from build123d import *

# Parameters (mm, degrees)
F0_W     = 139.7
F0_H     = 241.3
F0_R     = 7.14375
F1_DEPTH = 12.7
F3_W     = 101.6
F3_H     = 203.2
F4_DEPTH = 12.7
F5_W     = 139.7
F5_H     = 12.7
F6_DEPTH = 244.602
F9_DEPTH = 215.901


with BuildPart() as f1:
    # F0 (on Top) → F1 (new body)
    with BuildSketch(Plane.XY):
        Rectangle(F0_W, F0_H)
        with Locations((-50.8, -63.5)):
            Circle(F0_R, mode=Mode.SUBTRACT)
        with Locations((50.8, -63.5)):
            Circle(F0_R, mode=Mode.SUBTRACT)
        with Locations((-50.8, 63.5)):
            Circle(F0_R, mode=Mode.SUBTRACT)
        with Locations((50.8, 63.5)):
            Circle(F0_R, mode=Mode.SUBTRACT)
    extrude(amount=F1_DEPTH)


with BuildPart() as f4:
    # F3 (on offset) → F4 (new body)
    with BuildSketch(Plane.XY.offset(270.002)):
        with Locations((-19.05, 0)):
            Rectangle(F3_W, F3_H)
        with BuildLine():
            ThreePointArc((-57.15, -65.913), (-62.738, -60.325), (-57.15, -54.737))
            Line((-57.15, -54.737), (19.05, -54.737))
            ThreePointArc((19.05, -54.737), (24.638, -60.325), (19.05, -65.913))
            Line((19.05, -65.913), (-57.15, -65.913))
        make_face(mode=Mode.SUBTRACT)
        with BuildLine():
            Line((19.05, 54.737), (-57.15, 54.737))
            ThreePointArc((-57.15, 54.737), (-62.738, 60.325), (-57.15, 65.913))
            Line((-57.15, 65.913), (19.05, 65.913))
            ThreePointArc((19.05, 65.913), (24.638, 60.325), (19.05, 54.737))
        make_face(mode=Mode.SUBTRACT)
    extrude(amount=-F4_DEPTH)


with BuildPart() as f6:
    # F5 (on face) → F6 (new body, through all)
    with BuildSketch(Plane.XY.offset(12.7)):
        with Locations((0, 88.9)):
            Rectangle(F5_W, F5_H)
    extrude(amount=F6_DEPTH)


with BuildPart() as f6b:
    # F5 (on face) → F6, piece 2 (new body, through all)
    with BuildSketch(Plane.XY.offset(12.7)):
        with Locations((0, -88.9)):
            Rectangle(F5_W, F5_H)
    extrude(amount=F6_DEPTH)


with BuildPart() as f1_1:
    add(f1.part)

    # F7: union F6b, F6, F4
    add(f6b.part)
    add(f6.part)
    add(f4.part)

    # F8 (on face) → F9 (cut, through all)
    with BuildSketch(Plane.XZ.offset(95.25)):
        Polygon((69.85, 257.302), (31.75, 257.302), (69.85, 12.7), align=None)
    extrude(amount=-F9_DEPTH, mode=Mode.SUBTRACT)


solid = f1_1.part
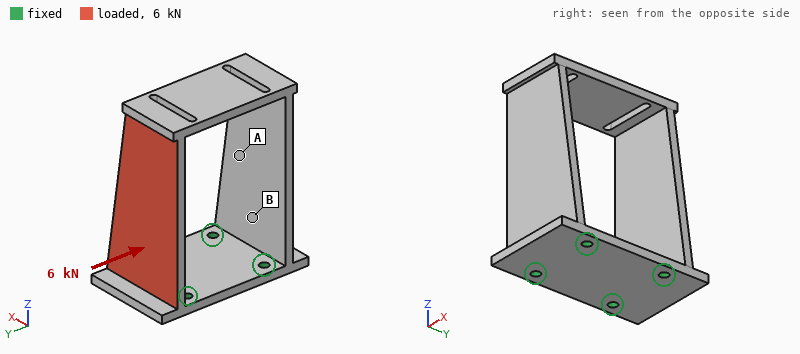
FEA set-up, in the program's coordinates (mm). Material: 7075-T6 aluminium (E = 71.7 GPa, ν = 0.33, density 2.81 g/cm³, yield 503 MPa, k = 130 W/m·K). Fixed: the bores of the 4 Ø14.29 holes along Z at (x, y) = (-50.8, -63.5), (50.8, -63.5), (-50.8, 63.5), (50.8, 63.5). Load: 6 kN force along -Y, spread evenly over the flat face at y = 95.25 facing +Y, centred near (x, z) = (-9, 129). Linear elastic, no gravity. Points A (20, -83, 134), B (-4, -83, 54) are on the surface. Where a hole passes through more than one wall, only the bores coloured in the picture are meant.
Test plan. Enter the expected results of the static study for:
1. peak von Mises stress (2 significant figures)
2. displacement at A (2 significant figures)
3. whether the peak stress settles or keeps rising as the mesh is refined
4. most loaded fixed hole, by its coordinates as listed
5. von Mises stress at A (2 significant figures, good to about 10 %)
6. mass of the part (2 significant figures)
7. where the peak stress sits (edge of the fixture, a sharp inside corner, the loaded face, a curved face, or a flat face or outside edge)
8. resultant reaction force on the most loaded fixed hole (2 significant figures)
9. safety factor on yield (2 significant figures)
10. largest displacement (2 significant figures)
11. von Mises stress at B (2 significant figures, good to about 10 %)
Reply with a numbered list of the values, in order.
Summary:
1. 290 MPa
2. 1.0 mm
3. settles
4. (-50.8, 63.5)
5. 17 MPa
6. 4.0 kg
7. a curved face
8. 2.6 kN
9. 1.8
10. 2.7 mm
11. 38 MPa
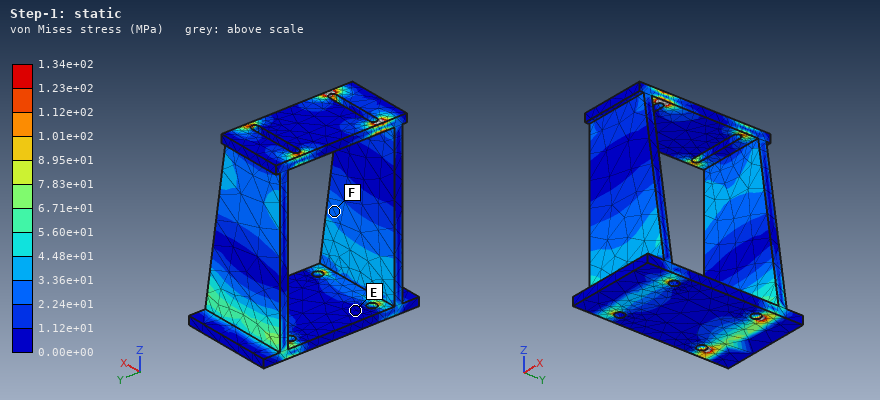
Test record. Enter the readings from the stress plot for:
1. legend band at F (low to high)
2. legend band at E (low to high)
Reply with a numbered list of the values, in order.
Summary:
1. 2.24e+01 to 3.36e+01 MPa
2. 0.00e+00 to 1.12e+01 MPa
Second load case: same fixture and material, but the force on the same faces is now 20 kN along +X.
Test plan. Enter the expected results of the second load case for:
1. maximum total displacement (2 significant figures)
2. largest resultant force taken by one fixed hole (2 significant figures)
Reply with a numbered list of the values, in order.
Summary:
1. 0.89 mm
2. 25 kN
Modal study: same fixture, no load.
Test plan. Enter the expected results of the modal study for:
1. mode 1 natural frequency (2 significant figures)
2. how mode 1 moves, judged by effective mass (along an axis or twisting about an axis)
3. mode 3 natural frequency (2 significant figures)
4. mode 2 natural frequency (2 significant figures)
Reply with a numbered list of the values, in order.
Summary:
1. 140 Hz
2. along Y
3. 630 Hz
4. 610 Hz
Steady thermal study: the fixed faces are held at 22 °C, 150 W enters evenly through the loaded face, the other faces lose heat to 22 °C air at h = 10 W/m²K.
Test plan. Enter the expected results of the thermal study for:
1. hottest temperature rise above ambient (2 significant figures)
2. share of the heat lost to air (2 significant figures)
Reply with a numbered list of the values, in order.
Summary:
1. 60 K
2. 25 %
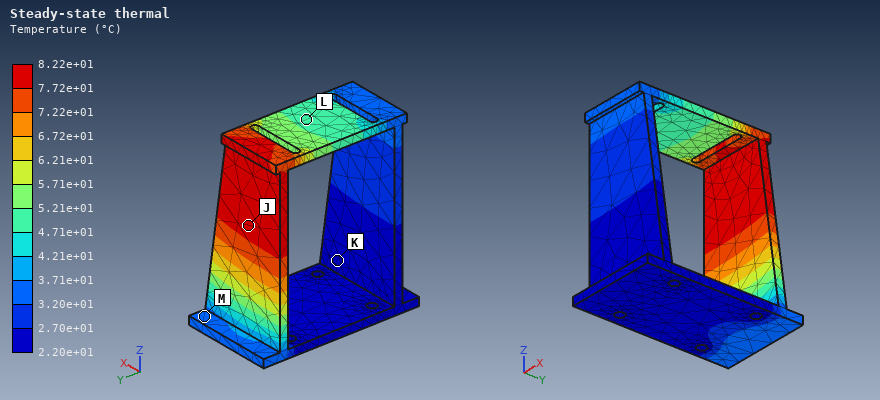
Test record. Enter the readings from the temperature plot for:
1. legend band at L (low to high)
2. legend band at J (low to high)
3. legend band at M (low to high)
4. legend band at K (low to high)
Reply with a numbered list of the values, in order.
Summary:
1. 4.71e+01 to 5.21e+01 °C
2. 7.72e+01 to 8.22e+01 °C
3. 3.20e+01 to 3.71e+01 °C
4. 2.20e+01 to 2.70e+01 °C
